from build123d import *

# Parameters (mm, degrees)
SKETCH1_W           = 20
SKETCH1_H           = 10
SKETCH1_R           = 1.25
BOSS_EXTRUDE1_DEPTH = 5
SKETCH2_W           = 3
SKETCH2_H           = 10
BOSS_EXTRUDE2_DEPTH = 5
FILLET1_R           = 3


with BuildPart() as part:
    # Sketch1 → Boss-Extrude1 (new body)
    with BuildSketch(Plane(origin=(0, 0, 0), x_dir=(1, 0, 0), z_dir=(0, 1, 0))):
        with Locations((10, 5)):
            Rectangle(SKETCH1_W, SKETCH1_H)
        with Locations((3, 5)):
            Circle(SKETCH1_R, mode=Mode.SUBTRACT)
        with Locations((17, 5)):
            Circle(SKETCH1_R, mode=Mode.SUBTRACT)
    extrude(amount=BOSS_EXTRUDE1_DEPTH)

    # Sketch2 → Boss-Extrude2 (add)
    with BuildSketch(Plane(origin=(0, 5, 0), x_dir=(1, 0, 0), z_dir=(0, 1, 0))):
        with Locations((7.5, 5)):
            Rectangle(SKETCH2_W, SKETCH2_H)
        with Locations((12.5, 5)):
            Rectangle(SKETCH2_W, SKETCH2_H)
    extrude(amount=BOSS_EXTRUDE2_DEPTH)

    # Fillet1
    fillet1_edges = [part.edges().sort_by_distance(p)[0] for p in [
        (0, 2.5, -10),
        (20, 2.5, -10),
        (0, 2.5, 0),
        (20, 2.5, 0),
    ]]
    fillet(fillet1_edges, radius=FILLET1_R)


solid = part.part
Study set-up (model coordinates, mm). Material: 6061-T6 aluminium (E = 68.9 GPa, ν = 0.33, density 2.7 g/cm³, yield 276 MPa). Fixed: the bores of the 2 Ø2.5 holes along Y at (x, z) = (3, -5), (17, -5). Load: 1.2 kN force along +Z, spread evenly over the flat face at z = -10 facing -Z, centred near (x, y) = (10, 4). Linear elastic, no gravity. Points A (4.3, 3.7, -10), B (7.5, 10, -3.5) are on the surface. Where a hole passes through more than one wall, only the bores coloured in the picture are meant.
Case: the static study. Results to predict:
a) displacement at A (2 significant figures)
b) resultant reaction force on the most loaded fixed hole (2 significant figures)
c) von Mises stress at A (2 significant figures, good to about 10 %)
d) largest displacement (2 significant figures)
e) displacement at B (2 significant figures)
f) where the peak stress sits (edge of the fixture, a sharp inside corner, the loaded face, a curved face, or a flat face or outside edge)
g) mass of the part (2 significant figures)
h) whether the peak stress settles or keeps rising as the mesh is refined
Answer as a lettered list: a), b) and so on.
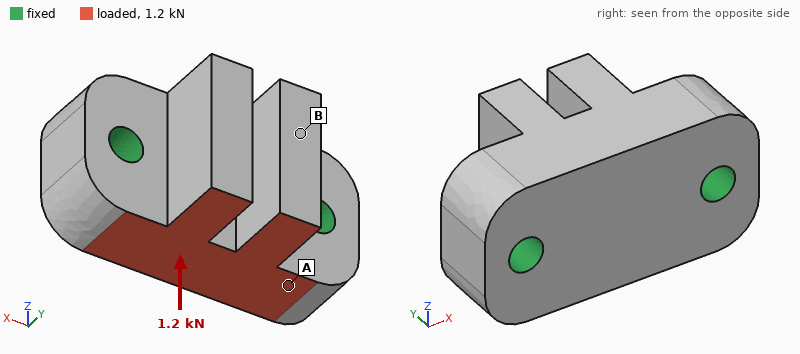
a) 2.5 µm
b) 610 N
c) 20 MPa
d) 8.6 µm
e) 6.9 µm
f) edge of the fixture
g) 3.3 g
h) keeps rising
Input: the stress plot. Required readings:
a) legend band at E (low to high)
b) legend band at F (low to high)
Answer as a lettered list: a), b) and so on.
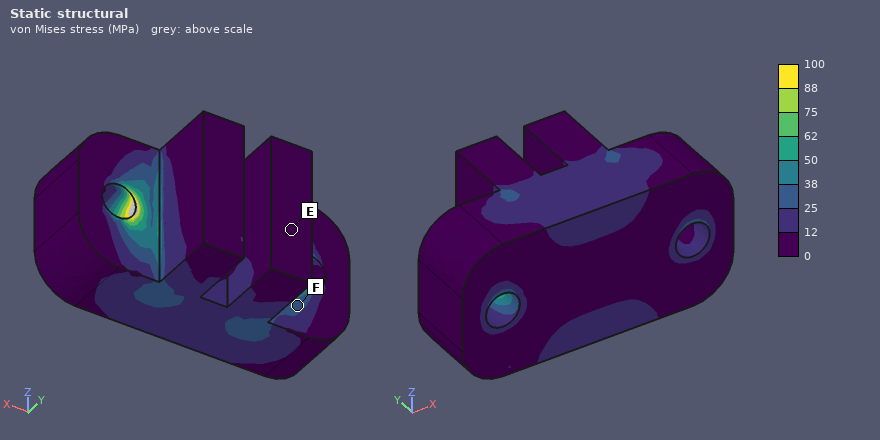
a) 0 to 12 MPa
b) 25 to 38 MPa
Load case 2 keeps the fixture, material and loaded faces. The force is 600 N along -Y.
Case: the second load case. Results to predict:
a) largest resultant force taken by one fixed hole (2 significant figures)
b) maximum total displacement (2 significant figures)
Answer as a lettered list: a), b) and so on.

a) 300 N
b) 9.2 µm
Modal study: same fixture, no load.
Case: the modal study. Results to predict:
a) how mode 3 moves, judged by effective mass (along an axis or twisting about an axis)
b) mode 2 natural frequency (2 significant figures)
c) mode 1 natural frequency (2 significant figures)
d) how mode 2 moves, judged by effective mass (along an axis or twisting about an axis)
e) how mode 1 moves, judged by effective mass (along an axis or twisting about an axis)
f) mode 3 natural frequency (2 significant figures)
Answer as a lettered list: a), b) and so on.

a) along X
b) 50 kHz
c) 42 kHz
d) along Y
e) along Z
f) 58 kHz
